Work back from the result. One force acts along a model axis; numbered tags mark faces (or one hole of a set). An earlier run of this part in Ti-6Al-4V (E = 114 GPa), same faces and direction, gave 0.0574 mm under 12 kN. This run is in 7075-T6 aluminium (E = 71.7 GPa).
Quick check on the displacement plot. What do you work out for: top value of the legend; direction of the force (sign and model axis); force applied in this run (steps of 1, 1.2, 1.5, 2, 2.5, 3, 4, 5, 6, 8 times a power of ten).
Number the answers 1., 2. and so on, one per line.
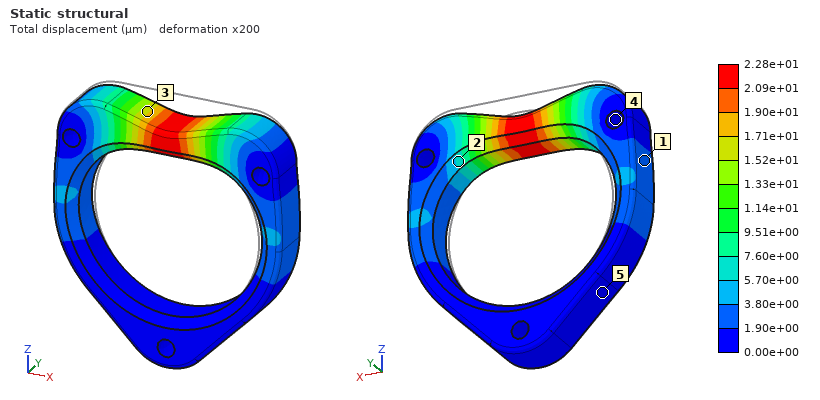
1. 2.28e+01 µm
2. -Z
3. 3 kN
